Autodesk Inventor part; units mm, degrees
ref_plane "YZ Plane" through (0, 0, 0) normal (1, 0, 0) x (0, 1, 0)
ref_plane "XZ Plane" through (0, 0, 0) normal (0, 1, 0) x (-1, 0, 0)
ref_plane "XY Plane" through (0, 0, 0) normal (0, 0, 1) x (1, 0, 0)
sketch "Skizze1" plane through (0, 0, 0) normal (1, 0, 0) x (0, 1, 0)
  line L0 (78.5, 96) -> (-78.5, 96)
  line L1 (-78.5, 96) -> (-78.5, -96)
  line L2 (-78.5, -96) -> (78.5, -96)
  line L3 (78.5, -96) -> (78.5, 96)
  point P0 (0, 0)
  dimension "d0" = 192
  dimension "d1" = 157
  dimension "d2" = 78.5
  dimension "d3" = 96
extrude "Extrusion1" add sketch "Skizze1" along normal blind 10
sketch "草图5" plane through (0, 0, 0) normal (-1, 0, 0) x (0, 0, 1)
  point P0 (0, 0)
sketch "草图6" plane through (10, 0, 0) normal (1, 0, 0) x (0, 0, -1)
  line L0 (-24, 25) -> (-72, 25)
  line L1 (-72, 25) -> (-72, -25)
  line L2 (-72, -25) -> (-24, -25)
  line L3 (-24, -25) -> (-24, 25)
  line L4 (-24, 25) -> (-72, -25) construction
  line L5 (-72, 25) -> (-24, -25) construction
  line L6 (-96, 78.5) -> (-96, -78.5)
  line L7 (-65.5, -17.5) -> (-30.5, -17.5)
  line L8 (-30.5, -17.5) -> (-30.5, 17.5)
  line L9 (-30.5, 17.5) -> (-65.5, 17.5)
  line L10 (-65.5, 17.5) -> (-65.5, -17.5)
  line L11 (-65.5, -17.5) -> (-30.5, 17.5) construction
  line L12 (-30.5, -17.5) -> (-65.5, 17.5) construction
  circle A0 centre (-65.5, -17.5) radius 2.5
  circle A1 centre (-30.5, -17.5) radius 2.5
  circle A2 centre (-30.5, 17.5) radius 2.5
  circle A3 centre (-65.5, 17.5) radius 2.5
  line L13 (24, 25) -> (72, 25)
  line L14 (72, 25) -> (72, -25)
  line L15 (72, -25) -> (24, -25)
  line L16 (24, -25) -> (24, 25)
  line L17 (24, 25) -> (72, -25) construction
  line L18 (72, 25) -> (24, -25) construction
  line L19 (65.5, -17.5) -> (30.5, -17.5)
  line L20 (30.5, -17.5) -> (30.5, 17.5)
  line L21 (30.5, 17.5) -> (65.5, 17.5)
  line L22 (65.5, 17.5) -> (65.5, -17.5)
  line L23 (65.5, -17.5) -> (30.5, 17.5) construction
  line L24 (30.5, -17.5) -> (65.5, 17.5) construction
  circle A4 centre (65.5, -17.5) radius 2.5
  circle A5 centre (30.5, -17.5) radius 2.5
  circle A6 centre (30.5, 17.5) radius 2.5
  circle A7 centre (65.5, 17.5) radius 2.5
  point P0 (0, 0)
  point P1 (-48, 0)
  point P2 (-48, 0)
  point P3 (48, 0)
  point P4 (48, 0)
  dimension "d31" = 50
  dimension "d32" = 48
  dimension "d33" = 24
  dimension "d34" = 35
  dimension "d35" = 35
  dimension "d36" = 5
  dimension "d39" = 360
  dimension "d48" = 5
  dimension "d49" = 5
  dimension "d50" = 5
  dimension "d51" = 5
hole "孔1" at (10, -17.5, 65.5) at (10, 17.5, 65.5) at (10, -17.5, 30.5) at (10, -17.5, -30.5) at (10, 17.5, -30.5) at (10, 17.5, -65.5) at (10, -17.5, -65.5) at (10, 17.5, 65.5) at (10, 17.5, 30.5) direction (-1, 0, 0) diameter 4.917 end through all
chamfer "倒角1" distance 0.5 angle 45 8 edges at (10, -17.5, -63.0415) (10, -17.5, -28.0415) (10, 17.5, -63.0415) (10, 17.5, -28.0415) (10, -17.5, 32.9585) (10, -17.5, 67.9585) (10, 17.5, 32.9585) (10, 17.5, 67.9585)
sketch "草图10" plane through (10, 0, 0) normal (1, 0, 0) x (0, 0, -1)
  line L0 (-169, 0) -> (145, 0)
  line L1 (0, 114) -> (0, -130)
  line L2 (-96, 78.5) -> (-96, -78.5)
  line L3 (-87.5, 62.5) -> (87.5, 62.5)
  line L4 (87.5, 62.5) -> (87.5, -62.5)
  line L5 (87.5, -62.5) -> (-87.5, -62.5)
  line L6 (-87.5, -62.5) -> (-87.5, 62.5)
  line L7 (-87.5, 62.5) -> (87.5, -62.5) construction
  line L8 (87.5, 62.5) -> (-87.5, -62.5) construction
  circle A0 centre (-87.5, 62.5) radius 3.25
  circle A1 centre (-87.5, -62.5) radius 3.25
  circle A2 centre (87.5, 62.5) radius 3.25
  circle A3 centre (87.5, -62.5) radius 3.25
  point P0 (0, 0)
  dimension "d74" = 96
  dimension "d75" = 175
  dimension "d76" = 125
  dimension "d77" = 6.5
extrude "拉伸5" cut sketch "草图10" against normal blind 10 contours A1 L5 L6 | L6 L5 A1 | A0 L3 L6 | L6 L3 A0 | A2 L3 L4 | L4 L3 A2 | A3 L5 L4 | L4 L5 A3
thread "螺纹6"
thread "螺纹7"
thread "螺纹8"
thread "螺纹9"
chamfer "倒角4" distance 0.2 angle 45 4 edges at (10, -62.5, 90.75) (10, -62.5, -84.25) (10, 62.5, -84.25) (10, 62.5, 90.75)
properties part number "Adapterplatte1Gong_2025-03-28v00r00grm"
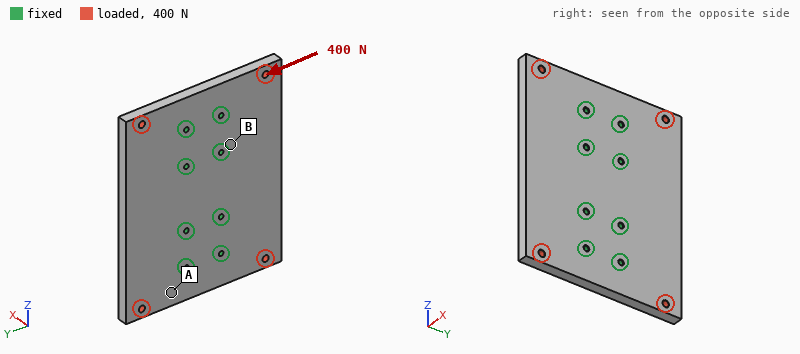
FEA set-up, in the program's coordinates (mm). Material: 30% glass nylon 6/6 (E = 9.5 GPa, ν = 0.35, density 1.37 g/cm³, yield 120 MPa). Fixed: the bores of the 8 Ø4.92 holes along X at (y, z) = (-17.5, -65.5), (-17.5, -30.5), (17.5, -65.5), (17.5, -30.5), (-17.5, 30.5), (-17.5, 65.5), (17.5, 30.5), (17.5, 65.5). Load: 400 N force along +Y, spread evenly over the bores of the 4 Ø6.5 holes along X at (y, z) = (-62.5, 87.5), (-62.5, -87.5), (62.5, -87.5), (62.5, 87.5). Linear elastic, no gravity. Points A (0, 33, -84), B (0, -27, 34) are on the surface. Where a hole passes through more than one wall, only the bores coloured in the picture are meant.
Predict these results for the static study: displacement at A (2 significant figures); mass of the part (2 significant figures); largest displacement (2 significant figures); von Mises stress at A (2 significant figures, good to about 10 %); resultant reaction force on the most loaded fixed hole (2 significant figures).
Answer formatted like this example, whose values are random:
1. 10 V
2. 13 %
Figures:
1. 1.4 µm
2. 410 g
3. 3.7 µm
4. 0.30 MPa
5. 91 N
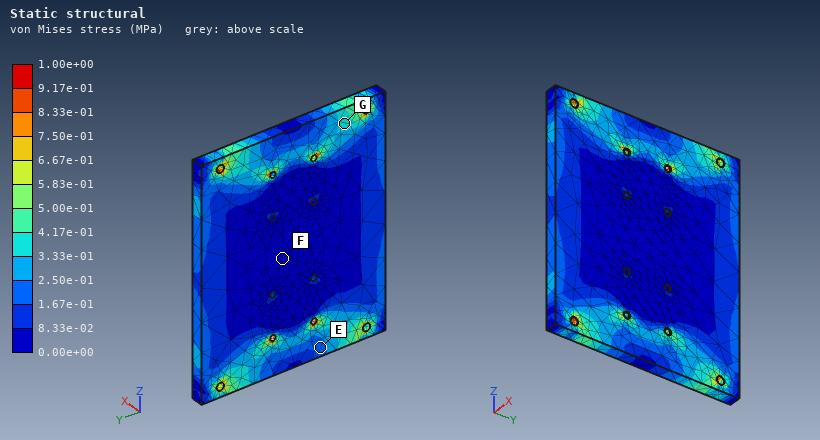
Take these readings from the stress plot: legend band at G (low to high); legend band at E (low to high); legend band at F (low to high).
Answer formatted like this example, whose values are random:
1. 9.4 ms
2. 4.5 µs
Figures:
1. 3.33e-01 to 4.17e-01 MPa
2. 1.67e-01 to 2.50e-01 MPa
3. 0.00e+00 to 8.33e-02 MPa
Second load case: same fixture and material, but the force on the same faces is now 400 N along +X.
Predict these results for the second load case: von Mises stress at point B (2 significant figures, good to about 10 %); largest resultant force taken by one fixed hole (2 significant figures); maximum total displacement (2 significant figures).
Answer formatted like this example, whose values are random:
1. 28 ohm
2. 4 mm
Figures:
1. 1.8 MPa
2. 120 N
3. 0.14 mm
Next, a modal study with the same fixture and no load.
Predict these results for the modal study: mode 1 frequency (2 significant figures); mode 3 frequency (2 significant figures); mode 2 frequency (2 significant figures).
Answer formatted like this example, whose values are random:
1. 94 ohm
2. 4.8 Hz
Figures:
1. 1000 Hz
2. 1300 Hz
3. 1000 Hz
